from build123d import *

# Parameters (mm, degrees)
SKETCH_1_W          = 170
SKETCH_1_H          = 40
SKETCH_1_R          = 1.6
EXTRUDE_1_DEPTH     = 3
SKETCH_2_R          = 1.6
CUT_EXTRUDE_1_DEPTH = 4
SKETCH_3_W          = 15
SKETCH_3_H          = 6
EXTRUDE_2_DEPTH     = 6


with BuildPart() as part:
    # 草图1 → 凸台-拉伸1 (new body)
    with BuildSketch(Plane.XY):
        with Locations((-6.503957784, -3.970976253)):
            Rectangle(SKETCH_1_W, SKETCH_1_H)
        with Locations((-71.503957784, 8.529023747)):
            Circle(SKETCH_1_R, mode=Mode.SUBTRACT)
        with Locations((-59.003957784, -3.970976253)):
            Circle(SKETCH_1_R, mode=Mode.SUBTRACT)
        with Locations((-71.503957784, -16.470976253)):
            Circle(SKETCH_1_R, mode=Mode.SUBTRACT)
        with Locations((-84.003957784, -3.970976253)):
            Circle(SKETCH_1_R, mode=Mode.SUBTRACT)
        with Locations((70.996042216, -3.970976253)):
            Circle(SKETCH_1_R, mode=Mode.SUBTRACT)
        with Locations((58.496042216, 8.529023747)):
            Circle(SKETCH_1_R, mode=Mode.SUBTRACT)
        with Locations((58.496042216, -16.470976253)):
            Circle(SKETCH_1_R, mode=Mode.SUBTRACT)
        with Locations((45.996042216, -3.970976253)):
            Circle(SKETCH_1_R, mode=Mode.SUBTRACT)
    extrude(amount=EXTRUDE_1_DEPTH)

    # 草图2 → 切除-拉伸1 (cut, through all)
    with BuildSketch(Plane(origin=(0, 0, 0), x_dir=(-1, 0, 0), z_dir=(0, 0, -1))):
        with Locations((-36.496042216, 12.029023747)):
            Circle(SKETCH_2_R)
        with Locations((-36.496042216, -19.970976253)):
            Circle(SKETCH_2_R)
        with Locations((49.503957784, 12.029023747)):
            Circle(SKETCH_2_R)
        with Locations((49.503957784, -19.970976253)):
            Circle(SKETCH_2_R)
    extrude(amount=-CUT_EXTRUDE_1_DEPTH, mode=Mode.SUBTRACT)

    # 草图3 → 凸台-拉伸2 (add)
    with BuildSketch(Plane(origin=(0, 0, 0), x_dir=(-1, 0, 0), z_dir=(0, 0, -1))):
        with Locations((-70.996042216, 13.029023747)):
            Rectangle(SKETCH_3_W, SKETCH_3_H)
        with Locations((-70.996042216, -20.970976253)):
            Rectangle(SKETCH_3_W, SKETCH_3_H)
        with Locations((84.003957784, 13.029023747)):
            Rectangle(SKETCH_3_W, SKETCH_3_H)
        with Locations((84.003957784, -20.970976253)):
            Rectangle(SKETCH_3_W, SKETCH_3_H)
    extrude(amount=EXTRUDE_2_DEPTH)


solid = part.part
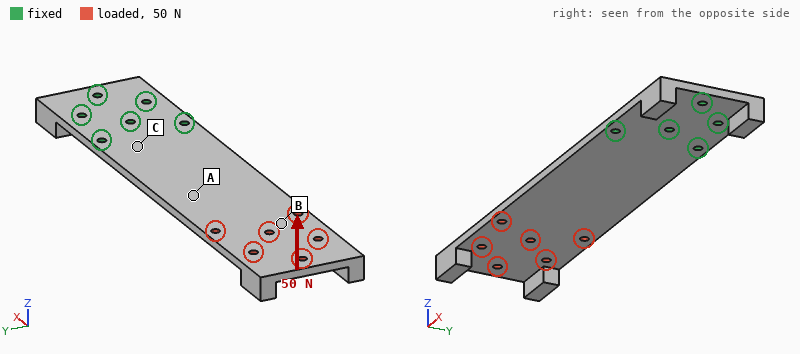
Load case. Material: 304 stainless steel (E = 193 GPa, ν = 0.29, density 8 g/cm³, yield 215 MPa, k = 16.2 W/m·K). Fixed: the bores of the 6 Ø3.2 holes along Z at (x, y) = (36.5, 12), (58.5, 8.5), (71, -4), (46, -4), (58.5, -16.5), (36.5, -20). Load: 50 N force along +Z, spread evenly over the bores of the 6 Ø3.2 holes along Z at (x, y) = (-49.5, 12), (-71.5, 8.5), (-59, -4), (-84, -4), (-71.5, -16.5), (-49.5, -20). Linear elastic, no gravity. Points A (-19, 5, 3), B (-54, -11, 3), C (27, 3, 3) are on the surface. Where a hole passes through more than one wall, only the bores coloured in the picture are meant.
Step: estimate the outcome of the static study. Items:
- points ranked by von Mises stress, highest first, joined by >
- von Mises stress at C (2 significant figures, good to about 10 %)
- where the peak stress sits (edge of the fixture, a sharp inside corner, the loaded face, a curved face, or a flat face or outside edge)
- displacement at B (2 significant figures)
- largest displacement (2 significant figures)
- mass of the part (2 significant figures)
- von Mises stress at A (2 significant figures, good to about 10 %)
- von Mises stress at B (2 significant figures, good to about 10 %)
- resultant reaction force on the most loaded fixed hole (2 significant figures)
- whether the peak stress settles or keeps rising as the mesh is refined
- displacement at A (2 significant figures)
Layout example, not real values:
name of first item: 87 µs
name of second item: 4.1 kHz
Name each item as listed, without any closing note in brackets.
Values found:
points ranked by von Mises stress, highest first, joined by >: C > A > B
von Mises stress at C: 70 MPa
where the peak stress sits: edge of the fixture
displacement at B: 0.85 mm
largest displacement: 1.4 mm
mass of the part: 180 g
von Mises stress at A: 37 MPa
von Mises stress at B: 11 MPa
resultant reaction force on the most loaded fixed hole: 100 N
whether the peak stress settles or keeps rising as the mesh is refined: keeps rising
displacement at A: 0.38 mm
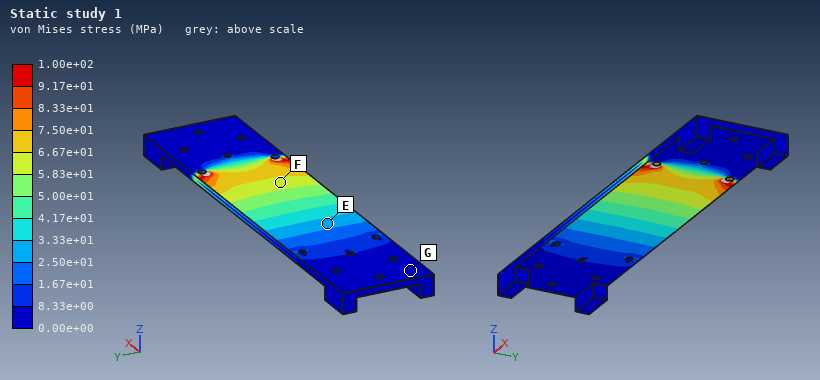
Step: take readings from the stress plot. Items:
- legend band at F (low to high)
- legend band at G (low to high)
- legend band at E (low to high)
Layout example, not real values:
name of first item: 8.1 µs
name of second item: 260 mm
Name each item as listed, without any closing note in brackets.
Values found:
legend band at F: 5.83e+01 to 6.67e+01 MPa
legend band at G: 0.00e+00 to 8.33e+00 MPa
legend band at E: 2.50e+01 to 3.33e+01 MPa
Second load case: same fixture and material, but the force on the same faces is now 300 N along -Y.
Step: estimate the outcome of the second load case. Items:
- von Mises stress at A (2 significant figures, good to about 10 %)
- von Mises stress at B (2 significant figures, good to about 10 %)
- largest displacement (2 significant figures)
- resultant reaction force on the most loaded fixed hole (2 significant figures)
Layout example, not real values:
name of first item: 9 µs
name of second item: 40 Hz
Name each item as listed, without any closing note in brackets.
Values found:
von Mises stress at A: 9.3 MPa
von Mises stress at B: 4.7 MPa
largest displacement: 53 µm
resultant reaction force on the most loaded fixed hole: 870 N
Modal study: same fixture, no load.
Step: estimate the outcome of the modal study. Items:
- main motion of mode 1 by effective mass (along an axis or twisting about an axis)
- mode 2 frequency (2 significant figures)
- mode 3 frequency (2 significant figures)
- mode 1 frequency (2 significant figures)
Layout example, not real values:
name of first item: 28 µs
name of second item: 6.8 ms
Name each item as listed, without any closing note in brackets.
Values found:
main motion of mode 1 by effective mass: along Z
mode 2 frequency: 820 Hz
mode 3 frequency: 840 Hz
mode 1 frequency: 130 Hz
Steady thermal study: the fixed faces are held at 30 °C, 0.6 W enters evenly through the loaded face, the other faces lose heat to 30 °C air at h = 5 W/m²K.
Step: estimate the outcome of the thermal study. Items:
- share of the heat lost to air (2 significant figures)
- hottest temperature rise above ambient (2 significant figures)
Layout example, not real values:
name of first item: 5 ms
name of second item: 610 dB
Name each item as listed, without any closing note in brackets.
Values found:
share of the heat lost to air: 71 %
hottest temperature rise above ambient: 13 K
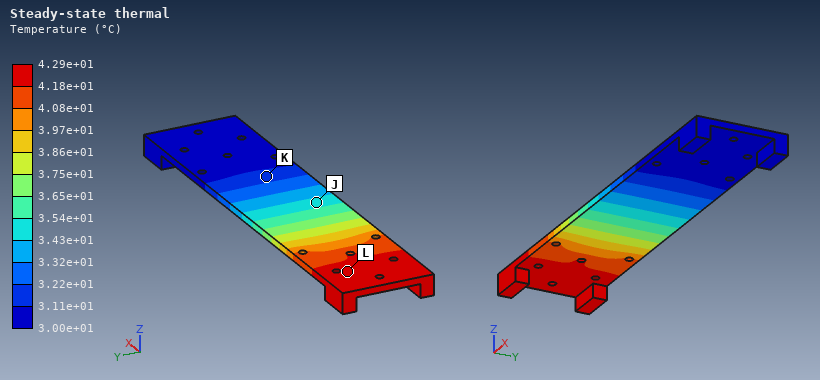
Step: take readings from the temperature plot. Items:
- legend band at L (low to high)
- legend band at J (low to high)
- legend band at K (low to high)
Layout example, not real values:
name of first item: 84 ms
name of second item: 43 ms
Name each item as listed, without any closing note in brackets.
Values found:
legend band at L: 4.18e+01 to 4.29e+01 °C
legend band at J: 3.43e+01 to 3.54e+01 °C
legend band at K: 3.11e+01 to 3.22e+01 °C
